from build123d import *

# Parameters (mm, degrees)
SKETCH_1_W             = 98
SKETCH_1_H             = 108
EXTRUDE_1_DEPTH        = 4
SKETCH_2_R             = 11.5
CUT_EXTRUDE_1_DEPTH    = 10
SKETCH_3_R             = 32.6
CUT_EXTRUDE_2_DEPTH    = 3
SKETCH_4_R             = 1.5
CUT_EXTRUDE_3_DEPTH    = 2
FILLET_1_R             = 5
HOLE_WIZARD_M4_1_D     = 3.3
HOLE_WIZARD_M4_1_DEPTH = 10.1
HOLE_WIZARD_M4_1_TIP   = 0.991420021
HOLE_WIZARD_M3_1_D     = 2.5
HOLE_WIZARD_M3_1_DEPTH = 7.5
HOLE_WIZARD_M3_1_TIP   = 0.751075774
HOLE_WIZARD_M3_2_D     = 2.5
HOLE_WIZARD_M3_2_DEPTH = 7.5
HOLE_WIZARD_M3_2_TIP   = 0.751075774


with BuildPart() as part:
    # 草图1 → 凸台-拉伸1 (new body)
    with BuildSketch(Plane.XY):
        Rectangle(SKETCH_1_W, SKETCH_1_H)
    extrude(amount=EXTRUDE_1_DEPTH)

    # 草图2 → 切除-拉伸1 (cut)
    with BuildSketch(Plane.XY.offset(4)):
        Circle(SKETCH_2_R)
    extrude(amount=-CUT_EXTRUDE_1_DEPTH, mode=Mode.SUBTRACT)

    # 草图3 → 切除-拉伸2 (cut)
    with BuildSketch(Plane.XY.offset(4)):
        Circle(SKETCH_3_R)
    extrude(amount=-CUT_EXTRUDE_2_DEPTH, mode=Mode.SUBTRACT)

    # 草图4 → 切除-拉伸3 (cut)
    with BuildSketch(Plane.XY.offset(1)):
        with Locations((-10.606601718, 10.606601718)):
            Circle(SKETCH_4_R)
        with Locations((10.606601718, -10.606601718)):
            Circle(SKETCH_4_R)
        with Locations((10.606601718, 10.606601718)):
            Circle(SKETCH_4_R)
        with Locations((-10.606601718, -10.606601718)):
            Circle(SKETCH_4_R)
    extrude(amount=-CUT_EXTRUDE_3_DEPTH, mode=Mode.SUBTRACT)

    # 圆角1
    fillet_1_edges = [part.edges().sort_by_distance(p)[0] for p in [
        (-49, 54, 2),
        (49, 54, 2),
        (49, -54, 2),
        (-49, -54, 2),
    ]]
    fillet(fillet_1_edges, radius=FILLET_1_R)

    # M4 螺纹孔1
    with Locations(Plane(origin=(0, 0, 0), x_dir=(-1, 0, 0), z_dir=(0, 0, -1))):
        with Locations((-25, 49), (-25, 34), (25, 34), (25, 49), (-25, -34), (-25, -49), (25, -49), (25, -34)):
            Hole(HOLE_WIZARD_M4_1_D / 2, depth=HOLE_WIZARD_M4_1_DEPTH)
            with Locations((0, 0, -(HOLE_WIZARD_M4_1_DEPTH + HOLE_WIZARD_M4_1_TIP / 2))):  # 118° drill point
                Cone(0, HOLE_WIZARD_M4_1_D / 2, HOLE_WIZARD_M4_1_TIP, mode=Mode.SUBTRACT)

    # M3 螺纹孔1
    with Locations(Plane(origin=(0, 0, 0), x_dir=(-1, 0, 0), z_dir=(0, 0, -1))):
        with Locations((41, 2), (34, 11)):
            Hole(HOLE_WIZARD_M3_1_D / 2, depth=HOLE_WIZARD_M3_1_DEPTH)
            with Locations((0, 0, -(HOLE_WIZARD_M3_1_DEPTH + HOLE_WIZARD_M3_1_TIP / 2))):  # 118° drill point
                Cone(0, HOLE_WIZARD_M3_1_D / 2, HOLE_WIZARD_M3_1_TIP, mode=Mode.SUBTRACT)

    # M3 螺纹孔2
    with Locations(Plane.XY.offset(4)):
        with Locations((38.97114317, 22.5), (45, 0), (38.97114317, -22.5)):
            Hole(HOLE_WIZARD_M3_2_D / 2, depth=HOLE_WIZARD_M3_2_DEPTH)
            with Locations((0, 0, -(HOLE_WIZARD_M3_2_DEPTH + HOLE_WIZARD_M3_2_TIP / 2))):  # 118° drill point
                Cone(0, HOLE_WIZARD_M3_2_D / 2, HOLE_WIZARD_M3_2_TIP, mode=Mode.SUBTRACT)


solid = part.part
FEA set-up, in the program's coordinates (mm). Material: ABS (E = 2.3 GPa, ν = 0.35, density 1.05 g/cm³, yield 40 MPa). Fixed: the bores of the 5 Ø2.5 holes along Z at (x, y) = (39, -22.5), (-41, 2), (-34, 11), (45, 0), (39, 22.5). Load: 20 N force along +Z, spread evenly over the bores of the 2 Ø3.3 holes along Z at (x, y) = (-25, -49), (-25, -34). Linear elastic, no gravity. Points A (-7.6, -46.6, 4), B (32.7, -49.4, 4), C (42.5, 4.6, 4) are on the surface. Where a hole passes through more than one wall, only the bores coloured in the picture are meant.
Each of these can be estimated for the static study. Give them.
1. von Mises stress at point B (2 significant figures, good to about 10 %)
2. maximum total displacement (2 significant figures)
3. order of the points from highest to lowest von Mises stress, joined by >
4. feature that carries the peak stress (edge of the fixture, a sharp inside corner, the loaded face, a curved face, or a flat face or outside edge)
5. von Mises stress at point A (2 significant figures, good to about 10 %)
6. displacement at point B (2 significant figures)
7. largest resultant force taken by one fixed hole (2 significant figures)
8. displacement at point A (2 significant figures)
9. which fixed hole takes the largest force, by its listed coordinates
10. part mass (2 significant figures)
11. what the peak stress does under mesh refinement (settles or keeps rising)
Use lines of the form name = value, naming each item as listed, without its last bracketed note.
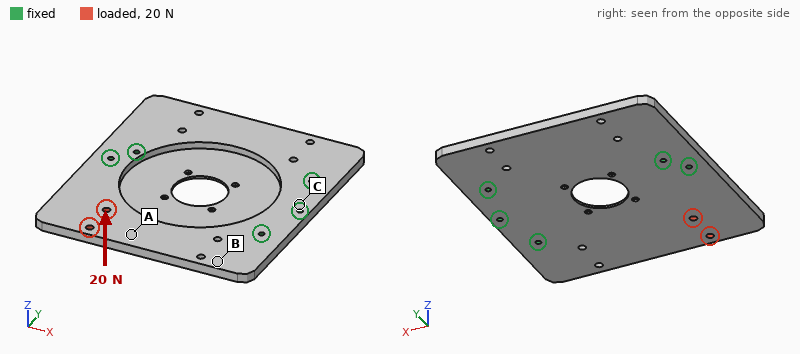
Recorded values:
von Mises stress at point B = 1.8 MPa
maximum total displacement = 1.4 mm
order of the points from highest to lowest von Mises stress, joined by > = A > B > C
feature that carries the peak stress = edge of the fixture
von Mises stress at point A = 2.2 MPa
displacement at point B = 0.25 mm
largest resultant force taken by one fixed hole = 37 N
displacement at point A = 0.87 mm
which fixed hole takes the largest force, by its listed coordinates = (-41, 2)
part mass = 33 g
what the peak stress does under mesh refinement = keeps rising
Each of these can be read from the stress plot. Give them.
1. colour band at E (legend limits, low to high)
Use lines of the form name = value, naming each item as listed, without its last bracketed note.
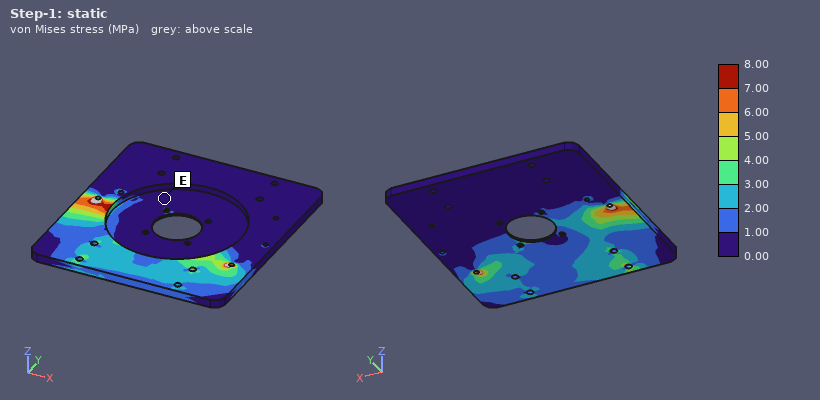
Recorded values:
colour band at E = 0.00 to 1.00 MPa
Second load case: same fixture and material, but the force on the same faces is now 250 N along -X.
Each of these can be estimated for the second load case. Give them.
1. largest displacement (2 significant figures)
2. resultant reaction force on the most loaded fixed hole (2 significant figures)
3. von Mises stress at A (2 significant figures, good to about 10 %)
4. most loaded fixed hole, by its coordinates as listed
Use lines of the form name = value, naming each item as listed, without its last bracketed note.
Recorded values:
largest displacement = 0.17 mm
resultant reaction force on the most loaded fixed hole = 170 N
von Mises stress at A = 2.4 MPa
most loaded fixed hole, by its coordinates as listed = (39, -22.5)
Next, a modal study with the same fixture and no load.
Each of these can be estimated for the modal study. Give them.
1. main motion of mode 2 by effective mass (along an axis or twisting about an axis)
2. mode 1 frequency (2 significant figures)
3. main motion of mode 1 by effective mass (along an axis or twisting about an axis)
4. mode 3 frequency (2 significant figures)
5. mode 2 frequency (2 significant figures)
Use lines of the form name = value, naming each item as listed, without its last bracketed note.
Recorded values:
main motion of mode 2 by effective mass = along Z
mode 1 frequency = 290 Hz
main motion of mode 1 by effective mass = along Z
mode 3 frequency = 720 Hz
mode 2 frequency = 410 Hz
